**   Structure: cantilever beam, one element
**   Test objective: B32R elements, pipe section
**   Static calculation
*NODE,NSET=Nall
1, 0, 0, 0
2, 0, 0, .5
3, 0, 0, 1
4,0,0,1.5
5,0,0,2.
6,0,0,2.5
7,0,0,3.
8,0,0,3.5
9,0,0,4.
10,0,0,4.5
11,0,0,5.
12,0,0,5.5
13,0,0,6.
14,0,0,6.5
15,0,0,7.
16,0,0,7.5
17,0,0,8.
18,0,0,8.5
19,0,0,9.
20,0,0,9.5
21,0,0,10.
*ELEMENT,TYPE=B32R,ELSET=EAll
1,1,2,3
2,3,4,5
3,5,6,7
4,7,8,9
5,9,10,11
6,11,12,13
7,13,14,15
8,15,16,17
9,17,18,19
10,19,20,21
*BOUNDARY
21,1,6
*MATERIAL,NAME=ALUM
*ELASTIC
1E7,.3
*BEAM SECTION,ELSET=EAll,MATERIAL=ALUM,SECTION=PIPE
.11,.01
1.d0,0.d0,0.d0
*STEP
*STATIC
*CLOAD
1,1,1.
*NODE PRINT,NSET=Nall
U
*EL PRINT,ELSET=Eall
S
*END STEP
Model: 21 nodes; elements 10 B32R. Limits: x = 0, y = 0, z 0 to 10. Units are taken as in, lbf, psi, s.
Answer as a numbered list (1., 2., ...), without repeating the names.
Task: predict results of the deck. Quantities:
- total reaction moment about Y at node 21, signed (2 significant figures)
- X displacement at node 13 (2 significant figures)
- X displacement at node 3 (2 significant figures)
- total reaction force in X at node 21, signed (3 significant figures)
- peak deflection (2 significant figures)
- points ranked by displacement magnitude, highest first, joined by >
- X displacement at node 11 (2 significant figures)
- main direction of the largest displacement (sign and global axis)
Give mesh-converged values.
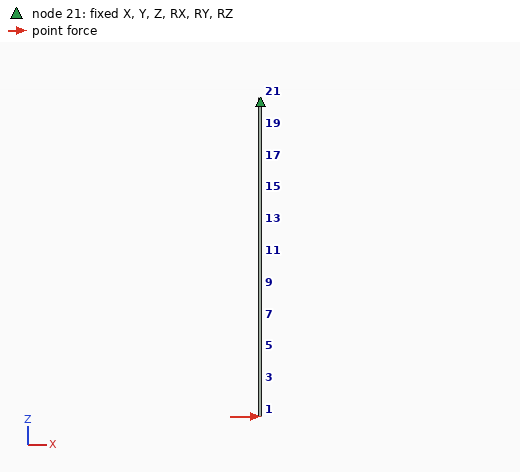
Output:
1. 10 lbf·in
2. 0.19 in
3. 0.78 in
4. -1.00 lbf
5. 0.92 in
6. node 3 > node 5 > node 7 > node 11 > node 13
7. 0.29 in
8. +X
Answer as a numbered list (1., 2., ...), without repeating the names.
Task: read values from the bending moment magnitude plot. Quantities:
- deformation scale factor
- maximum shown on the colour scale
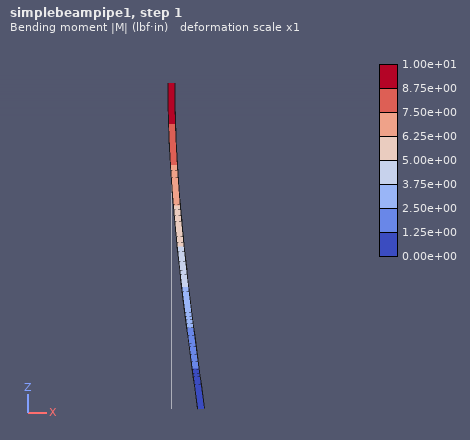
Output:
1. 1
2. 1.00e+01 lbf·in
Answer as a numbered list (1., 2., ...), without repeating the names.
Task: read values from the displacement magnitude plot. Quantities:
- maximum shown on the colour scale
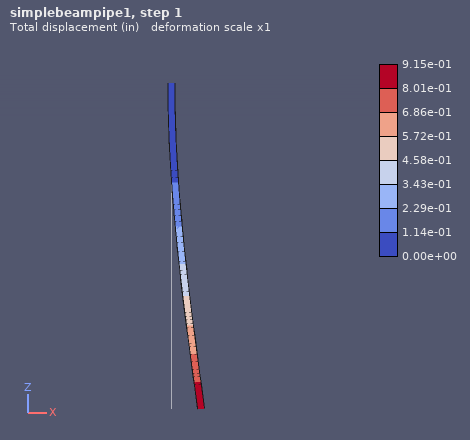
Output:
1. 9.15e-01 in
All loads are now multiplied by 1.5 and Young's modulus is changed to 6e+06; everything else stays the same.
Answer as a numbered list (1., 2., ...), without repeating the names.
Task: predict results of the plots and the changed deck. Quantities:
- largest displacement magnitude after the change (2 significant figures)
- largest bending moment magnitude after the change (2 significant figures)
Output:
1. 2.3 in
2. 15 lbf·in
